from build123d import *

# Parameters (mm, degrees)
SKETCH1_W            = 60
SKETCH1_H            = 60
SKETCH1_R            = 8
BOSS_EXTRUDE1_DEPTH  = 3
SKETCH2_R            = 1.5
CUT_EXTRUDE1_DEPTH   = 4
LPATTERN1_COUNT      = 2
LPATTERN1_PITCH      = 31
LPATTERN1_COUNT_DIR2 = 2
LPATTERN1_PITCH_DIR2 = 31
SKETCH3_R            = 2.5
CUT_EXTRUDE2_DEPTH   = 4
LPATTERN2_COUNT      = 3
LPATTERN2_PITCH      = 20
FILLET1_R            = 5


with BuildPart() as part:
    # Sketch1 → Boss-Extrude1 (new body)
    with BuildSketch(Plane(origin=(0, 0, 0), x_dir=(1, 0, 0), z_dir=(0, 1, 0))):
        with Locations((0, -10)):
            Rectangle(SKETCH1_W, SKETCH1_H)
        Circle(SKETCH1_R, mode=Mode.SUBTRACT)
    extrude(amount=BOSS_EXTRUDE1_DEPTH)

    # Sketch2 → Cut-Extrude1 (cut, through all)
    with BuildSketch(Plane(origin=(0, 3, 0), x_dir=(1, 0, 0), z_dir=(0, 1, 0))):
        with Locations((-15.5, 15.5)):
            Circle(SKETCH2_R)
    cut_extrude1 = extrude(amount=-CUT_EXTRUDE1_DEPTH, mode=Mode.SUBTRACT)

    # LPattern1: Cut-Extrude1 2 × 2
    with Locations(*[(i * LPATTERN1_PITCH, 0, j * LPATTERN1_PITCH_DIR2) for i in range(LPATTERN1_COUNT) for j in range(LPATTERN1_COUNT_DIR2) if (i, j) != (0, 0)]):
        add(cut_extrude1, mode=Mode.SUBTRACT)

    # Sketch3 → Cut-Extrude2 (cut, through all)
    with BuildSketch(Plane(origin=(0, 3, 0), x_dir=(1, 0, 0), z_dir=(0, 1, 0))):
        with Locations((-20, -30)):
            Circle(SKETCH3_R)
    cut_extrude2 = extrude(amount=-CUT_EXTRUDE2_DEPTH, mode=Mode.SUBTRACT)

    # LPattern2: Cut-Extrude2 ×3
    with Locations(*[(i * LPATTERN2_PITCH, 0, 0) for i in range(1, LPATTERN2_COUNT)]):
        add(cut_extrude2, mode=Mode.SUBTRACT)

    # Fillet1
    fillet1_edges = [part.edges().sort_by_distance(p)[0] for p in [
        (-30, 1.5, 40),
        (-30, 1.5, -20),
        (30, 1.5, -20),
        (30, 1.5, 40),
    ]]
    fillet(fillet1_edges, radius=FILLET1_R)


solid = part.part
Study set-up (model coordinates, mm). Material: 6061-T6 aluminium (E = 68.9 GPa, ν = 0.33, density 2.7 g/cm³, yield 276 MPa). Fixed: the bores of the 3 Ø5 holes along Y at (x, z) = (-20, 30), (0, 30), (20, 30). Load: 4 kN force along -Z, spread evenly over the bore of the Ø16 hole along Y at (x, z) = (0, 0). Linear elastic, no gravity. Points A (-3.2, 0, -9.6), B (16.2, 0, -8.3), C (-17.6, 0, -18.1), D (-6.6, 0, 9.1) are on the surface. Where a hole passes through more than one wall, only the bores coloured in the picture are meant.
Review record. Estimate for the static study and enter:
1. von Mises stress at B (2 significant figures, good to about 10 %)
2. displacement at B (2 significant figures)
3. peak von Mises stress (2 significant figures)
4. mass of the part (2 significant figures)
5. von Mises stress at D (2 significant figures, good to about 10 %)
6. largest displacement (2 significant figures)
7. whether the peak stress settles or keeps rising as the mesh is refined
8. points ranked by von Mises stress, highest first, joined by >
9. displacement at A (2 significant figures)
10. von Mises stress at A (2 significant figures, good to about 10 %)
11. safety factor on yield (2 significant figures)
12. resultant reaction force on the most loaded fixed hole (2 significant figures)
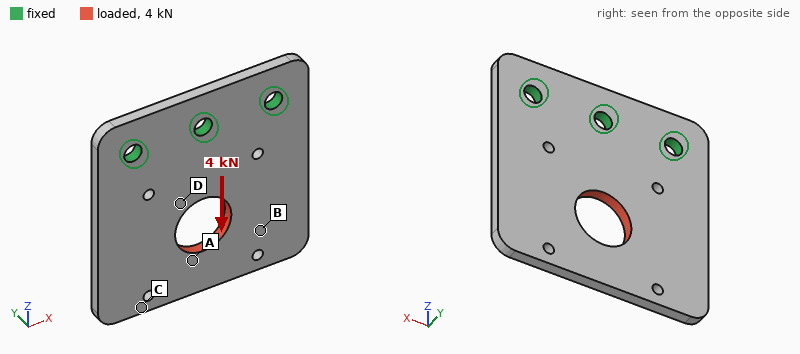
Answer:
13 MPa
12 µm
84 MPa
27 g
42 MPa
25 µm
settles
D > A > B > C
23 µm
25 MPa
3.3
1.4 kN
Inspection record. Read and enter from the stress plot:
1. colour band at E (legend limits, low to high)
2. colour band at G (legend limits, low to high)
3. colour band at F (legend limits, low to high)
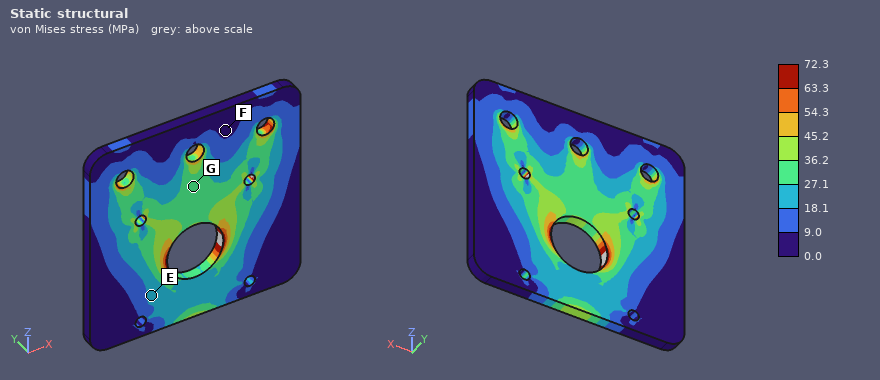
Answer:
18.1 to 27.1 MPa
27.1 to 36.2 MPa
0.0 to 9.0 MPa
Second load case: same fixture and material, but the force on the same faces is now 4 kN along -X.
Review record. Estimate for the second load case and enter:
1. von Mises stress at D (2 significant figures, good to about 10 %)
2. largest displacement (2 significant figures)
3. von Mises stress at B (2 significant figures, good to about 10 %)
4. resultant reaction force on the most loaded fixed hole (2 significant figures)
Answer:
54 MPa
77 µm
17 MPa
3.0 kN
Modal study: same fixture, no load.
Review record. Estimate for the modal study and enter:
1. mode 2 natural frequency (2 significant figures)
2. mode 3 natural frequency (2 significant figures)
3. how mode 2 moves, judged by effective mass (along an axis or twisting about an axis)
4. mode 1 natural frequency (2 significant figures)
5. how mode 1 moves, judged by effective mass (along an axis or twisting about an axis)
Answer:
2100 Hz
5200 Hz
twisting about Z
1100 Hz
along Y
